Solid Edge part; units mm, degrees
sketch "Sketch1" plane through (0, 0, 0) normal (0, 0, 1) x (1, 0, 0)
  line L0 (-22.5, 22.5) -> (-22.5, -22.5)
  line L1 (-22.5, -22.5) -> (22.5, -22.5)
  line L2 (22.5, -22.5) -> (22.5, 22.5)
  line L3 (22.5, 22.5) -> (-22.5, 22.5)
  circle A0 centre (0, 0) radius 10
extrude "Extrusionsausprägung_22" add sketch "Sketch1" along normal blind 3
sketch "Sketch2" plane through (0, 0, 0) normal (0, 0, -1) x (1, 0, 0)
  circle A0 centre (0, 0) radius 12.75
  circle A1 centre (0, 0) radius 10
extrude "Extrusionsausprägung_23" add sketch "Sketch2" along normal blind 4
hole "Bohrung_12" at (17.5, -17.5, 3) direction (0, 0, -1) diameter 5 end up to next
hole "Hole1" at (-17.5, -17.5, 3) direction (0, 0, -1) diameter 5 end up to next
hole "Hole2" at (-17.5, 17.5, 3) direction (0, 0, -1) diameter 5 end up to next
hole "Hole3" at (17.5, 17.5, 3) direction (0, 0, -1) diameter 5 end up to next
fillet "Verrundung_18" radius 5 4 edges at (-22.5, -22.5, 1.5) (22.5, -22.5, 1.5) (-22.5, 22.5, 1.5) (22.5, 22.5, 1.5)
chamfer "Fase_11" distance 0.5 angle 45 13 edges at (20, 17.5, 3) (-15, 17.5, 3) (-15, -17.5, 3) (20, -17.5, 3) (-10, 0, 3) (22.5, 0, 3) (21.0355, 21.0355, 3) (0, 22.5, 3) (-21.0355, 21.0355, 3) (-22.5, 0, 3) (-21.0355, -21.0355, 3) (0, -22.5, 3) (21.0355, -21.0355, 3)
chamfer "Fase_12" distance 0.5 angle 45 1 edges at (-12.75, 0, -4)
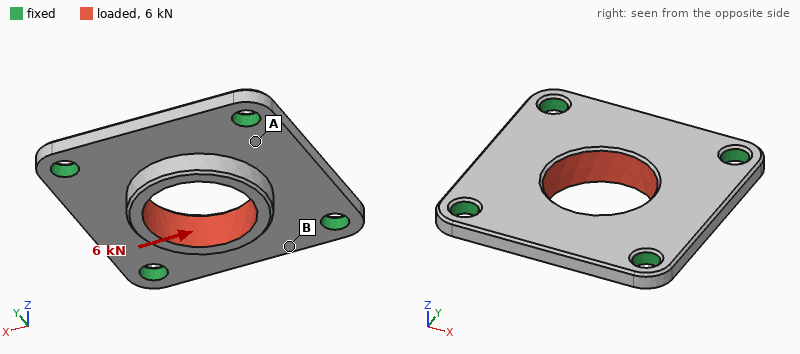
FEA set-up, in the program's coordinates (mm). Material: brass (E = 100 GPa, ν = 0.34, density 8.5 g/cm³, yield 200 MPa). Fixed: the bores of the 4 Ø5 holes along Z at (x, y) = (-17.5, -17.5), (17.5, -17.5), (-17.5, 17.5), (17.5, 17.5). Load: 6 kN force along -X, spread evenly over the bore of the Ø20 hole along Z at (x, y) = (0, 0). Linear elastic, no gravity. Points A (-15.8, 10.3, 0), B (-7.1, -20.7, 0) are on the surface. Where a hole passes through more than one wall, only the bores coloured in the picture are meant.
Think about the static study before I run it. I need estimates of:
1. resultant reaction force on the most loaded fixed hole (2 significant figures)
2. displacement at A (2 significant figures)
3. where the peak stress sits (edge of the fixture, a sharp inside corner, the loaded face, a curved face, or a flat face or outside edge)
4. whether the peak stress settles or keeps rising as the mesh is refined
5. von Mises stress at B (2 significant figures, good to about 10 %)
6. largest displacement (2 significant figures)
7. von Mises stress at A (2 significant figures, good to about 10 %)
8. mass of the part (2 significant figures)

1.6 kN
6.9 µm
edge of the fixture
keeps rising
26 MPa
22 µm
46 MPa
47 g
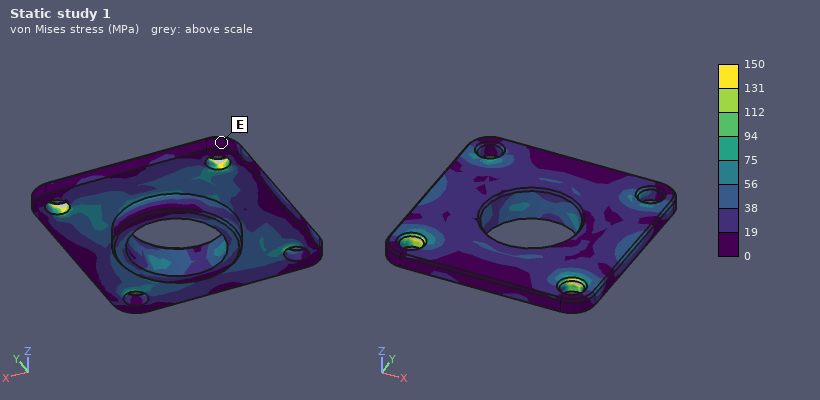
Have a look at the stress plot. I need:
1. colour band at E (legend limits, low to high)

0 to 19 MPa
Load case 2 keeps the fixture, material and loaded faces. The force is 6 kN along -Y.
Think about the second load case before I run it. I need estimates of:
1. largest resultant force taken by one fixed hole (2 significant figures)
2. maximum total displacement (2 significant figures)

1.6 kN
21 µm
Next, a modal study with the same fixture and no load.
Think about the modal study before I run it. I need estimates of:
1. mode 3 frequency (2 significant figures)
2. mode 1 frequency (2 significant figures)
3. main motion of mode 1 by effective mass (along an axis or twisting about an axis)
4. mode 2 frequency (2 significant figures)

10 kHz
8200 Hz
along Z
10 kHz
